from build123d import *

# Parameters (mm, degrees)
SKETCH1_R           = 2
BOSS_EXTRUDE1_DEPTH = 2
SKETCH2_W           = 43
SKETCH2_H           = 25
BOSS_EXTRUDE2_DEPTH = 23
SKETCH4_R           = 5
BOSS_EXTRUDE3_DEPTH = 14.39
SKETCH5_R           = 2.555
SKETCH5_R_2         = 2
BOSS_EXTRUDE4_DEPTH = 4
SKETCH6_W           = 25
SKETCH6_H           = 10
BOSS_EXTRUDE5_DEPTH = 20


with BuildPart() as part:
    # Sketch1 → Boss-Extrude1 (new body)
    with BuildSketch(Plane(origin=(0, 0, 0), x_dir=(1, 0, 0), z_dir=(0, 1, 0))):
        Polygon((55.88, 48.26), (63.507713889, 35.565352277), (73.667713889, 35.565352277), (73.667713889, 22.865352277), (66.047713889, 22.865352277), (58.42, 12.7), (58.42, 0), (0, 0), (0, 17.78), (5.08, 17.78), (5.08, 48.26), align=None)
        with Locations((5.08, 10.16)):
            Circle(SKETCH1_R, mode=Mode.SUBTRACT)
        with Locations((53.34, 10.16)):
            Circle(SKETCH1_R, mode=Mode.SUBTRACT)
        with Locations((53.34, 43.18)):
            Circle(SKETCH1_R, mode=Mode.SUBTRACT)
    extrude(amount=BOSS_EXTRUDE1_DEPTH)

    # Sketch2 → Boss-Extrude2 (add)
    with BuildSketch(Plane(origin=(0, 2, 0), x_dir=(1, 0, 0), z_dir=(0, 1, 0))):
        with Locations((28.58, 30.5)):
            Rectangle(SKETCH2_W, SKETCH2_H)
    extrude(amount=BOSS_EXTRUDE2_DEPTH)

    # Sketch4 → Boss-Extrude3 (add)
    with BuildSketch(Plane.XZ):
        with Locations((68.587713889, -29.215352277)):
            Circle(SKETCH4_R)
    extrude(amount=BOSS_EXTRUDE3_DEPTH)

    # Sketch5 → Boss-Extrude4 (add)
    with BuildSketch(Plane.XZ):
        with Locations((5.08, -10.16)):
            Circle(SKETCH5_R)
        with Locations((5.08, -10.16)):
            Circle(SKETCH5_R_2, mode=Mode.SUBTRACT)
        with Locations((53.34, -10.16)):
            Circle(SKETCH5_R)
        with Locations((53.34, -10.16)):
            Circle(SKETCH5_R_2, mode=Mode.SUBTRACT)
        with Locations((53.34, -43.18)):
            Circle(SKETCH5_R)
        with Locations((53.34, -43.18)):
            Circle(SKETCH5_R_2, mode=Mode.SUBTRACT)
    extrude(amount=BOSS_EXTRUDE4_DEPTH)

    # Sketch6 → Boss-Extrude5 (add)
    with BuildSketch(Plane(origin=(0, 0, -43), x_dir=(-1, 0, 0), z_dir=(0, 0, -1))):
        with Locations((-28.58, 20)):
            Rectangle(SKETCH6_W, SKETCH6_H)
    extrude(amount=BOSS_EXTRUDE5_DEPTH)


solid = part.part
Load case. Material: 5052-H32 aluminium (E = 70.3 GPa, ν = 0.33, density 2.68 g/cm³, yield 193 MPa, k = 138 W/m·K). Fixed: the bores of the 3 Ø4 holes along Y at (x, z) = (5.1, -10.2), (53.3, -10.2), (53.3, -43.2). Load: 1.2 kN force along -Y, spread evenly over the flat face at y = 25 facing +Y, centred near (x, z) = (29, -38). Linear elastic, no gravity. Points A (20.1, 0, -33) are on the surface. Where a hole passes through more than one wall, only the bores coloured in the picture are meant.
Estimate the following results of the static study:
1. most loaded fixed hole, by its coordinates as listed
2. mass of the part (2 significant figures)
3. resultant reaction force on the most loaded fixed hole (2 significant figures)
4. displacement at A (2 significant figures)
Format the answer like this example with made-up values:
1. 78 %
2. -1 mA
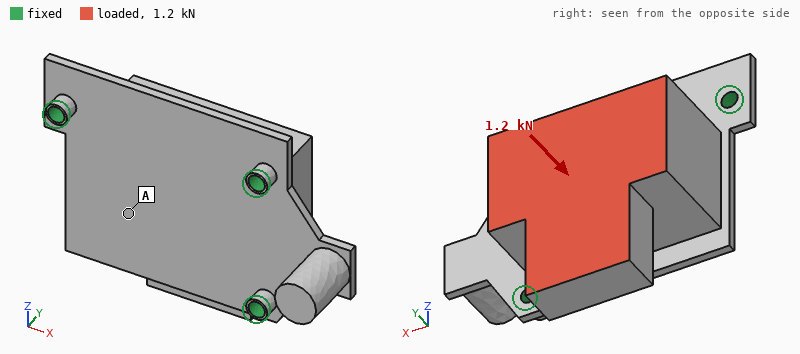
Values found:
1. (53.3, -43.2)
2. 98 g
3. 1.1 kN
4. 0.081 mm
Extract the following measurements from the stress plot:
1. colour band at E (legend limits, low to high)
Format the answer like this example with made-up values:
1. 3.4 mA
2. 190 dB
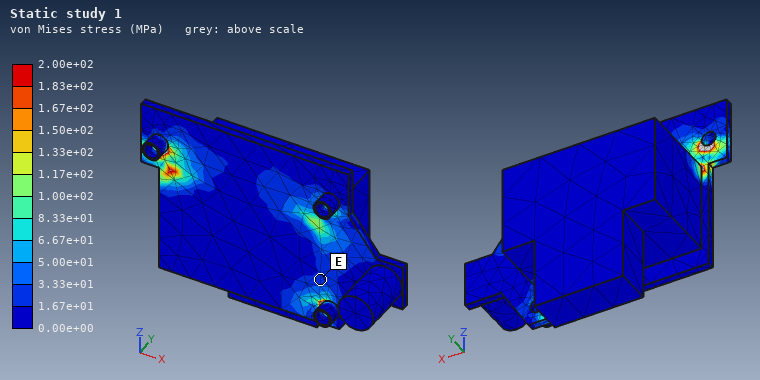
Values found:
1. 1.67e+01 to 3.33e+01 MPa
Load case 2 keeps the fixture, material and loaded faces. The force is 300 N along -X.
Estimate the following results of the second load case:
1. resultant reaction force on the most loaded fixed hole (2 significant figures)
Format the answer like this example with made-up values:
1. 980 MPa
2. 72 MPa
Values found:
1. 210 N
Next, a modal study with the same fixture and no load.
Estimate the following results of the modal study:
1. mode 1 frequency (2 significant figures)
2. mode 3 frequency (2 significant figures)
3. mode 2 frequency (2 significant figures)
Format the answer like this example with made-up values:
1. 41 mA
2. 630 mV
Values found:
1. 1600 Hz
2. 3200 Hz
3. 1800 Hz
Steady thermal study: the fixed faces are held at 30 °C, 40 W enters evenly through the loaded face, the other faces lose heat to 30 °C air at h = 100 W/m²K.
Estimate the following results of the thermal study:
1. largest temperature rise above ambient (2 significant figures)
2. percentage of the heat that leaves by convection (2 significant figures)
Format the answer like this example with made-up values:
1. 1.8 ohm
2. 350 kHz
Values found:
1. 28 K
2. 39 %
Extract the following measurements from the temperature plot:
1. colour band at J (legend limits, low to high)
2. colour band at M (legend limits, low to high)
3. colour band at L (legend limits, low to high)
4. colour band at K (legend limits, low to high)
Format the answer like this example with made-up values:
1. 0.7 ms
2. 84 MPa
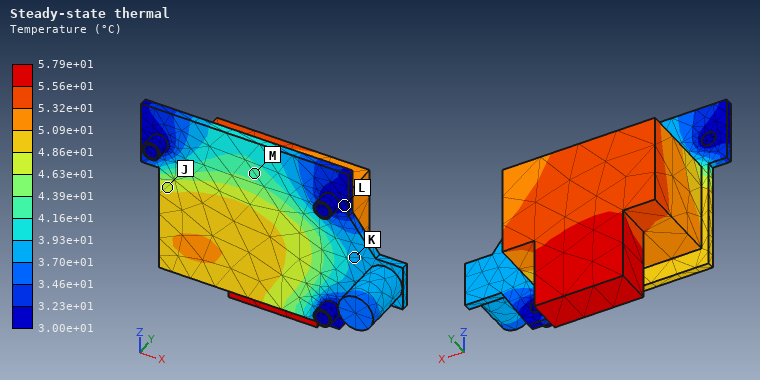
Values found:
1. 4.63e+01 to 4.86e+01 °C
2. 4.16e+01 to 4.39e+01 °C
3. 3.00e+01 to 3.23e+01 °C
4. 3.70e+01 to 3.93e+01 °C
